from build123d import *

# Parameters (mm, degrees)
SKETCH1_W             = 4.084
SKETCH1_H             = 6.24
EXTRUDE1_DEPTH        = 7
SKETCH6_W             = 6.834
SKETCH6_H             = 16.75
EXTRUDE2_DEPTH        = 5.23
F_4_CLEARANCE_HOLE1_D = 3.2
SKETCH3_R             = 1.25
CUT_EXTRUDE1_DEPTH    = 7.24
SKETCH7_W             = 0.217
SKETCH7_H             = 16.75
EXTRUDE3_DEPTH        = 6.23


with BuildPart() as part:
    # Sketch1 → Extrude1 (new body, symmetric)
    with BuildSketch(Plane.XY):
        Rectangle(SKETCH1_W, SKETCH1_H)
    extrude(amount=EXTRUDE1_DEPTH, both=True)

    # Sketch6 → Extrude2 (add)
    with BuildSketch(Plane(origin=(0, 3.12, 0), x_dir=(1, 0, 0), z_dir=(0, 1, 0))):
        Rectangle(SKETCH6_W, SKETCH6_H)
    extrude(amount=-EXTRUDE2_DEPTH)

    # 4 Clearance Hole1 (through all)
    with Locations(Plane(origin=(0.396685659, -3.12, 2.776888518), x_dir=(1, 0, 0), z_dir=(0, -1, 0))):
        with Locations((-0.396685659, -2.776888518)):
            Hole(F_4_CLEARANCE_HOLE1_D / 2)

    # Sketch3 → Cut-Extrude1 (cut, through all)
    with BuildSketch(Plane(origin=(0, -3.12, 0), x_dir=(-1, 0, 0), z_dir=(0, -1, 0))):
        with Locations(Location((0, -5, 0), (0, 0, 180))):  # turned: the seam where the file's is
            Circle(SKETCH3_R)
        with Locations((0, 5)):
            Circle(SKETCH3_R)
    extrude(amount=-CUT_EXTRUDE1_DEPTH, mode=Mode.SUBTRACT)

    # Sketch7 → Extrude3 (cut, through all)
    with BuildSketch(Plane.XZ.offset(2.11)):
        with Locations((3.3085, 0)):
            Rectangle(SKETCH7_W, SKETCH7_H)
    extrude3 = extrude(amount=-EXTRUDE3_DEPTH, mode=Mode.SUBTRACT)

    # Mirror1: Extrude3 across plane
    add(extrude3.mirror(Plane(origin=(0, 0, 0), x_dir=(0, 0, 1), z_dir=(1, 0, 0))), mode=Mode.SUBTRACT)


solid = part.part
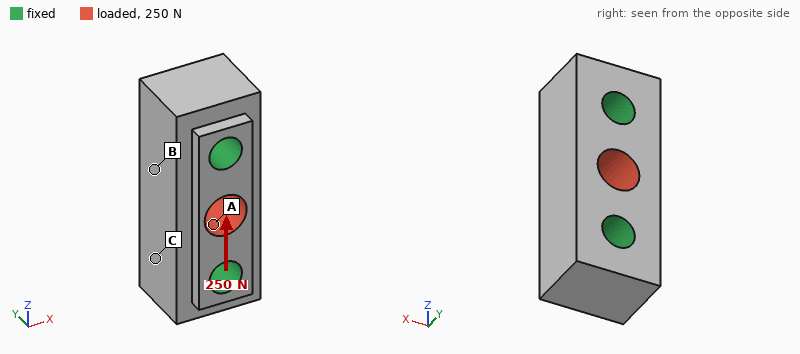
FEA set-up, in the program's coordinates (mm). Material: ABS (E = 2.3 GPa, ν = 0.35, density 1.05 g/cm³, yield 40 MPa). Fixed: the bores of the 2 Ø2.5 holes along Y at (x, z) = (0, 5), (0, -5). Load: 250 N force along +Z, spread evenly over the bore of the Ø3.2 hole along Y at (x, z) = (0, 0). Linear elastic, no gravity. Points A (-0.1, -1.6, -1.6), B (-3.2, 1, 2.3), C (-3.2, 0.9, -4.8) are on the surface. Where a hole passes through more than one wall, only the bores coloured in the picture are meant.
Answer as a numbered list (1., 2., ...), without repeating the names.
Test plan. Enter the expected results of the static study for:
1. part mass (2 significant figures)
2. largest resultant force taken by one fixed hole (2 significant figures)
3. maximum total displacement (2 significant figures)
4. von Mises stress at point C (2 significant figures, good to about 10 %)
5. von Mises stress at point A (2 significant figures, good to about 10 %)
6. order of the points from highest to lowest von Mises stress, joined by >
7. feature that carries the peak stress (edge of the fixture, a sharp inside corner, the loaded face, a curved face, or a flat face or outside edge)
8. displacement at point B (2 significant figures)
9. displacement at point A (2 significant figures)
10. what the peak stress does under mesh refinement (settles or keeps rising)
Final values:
1. 0.53 g
2. 130 N
3. 8.8 µm
4. 1.4 MPa
5. 5.6 MPa
6. A > C > B
7. edge of the fixture
8. 4.3 µm
9. 4.7 µm
10. keeps rising
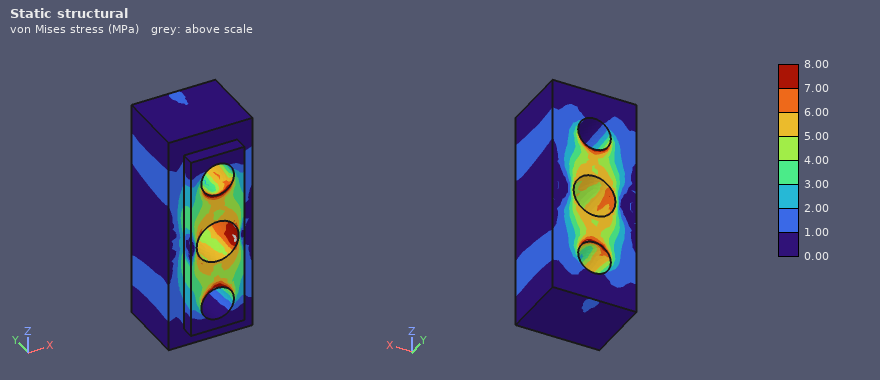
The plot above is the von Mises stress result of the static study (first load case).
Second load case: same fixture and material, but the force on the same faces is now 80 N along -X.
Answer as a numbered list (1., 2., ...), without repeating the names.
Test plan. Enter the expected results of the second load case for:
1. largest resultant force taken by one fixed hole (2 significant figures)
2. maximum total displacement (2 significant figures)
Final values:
1. 40 N
2. 12 µm
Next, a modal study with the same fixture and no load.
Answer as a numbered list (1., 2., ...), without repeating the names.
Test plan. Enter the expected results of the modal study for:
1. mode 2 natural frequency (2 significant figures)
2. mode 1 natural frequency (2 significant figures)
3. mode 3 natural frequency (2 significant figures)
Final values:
1. 49 kHz
2. 46 kHz
3. 49 kHz
